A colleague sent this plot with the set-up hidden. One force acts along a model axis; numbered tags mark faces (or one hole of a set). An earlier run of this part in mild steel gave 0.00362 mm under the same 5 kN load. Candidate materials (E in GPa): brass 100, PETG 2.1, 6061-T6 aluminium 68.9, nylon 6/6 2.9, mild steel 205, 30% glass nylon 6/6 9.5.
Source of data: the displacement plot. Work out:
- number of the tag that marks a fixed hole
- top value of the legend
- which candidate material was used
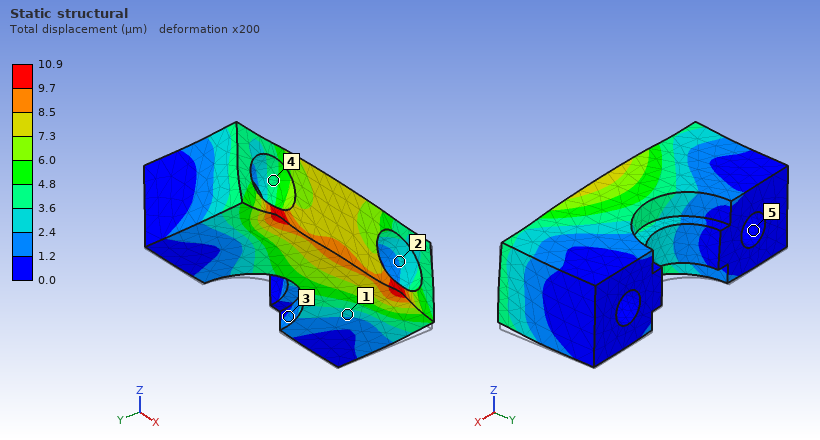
5
10.9 µm
6061-T6 aluminium
